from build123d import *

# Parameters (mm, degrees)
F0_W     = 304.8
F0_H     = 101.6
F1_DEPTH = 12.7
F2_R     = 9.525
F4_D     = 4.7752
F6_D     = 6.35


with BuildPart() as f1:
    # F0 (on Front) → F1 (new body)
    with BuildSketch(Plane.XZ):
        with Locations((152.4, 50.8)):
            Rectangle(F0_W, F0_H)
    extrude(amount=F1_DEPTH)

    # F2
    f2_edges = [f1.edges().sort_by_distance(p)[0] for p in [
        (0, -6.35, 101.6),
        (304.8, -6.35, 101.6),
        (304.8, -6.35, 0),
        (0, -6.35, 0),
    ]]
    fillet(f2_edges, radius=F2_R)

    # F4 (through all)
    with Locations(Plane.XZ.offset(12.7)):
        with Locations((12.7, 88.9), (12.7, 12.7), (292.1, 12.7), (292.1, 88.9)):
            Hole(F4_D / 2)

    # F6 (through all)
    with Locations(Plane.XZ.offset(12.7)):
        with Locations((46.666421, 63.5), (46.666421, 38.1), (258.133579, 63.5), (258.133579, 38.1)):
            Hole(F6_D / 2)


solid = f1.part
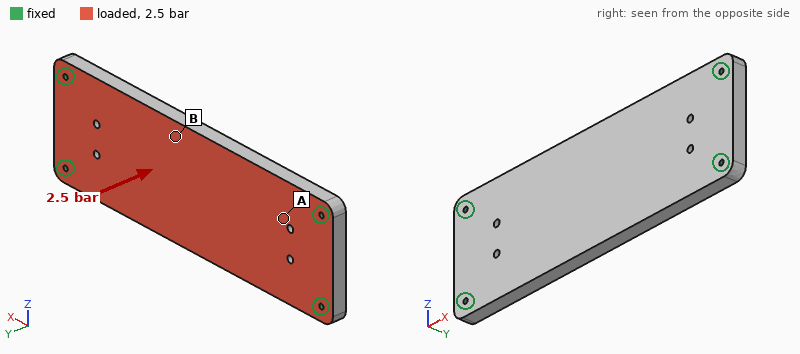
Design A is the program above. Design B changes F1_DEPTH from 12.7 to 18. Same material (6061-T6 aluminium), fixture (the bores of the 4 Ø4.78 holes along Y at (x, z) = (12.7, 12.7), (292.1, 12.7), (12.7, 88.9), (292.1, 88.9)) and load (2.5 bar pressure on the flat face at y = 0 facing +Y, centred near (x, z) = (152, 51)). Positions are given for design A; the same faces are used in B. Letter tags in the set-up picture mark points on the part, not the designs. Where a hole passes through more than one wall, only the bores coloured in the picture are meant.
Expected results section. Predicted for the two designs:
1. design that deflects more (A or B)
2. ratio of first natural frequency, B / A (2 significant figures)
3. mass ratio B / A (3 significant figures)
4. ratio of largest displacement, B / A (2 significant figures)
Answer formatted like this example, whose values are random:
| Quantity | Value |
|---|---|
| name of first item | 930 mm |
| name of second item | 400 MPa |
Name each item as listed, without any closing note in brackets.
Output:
| Quantity | Value |
|---|---|
| design that deflects more | A |
| ratio of first natural frequency, B / A | 1.4 |
| mass ratio B / A | 1.42 |
| ratio of largest displacement, B / A | 0.38 |
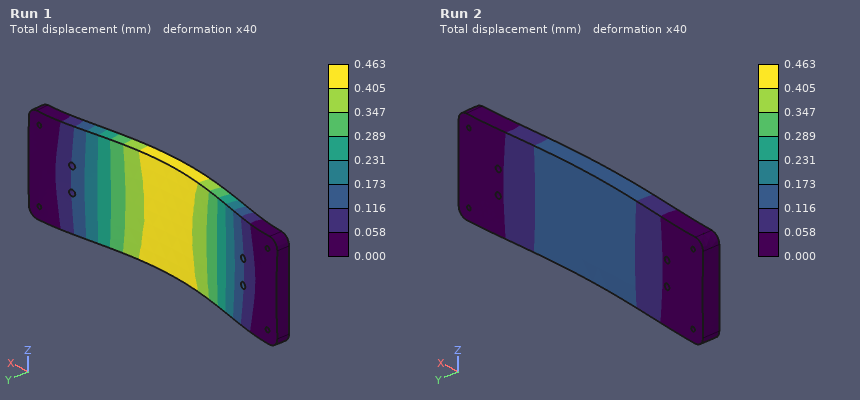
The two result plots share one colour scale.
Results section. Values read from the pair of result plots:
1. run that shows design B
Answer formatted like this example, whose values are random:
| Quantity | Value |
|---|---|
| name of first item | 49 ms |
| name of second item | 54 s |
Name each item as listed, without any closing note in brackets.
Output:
| Quantity | Value |
|---|---|
| run that shows design B | Run 2 |
